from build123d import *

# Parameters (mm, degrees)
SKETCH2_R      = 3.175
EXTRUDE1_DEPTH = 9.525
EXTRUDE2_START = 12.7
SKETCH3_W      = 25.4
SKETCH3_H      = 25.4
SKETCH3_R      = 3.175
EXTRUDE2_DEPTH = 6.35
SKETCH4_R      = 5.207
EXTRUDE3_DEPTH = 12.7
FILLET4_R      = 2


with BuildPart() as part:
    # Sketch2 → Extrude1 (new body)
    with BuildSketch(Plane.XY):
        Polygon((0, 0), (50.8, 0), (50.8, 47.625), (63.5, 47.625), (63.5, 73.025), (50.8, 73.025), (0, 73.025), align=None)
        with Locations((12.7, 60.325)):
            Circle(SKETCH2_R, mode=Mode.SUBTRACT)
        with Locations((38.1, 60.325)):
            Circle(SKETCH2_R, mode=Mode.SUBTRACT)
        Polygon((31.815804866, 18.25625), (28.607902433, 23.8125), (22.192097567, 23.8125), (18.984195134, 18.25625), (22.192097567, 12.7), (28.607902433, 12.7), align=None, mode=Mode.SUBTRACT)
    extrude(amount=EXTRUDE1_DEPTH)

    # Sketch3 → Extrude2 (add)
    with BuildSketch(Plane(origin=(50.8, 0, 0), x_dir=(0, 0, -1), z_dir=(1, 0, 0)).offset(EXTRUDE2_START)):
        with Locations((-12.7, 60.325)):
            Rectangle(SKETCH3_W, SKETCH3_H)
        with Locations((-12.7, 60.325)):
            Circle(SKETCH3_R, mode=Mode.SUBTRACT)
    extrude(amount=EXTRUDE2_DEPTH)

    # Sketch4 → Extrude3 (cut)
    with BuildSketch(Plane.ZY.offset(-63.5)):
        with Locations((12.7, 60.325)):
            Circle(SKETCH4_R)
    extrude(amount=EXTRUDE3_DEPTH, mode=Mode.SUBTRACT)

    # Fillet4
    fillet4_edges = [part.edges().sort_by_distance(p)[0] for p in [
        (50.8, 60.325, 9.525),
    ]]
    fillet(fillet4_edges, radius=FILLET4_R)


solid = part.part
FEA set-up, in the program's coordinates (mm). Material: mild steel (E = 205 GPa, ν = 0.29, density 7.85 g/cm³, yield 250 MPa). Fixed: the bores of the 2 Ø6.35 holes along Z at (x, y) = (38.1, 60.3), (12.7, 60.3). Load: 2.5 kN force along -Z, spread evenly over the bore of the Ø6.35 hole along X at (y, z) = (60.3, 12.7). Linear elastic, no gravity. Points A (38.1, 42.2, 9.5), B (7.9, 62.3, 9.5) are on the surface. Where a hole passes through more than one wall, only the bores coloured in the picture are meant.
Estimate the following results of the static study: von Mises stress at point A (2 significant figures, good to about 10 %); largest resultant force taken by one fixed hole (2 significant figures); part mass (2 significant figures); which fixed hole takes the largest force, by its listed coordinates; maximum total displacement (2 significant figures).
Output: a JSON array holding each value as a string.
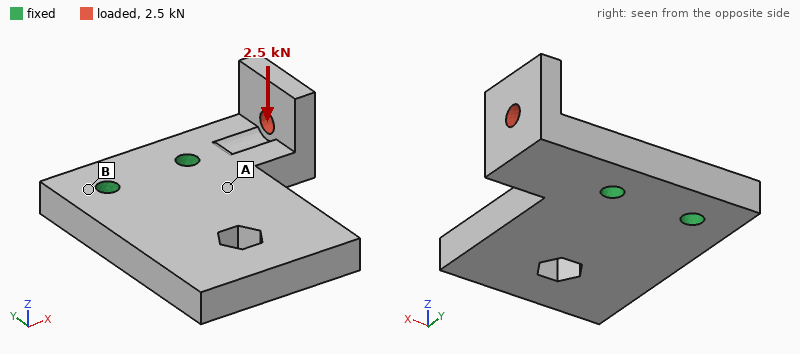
["32 MPa", "3.3 kN", "320 g", "(38.1, 60.3)", "82 µm"]
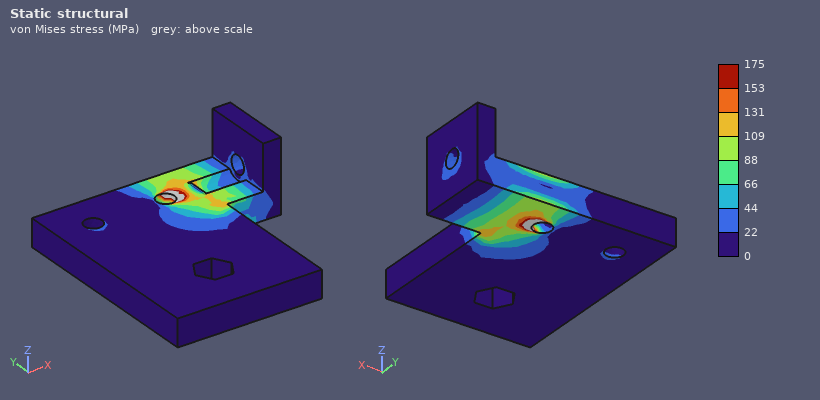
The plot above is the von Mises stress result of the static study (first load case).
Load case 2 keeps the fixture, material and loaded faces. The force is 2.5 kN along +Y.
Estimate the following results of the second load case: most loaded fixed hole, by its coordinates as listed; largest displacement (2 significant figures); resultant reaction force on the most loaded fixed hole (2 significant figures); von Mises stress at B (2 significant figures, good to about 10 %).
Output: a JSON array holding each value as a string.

["(38.1, 60.3)", "43 µm", "4.4 kN", "9.7 MPa"]
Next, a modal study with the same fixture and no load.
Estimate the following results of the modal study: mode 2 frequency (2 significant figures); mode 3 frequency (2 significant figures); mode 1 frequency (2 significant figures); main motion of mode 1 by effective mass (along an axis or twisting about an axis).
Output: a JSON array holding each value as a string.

["4900 Hz", "5400 Hz", "2200 Hz", "along Z"]
